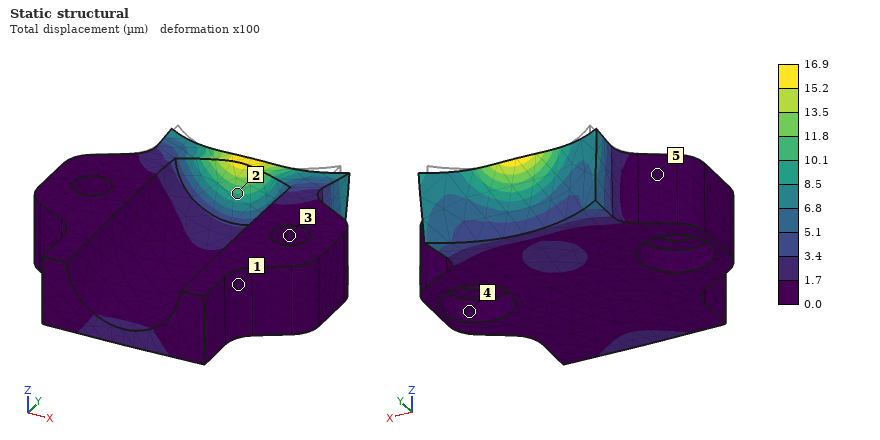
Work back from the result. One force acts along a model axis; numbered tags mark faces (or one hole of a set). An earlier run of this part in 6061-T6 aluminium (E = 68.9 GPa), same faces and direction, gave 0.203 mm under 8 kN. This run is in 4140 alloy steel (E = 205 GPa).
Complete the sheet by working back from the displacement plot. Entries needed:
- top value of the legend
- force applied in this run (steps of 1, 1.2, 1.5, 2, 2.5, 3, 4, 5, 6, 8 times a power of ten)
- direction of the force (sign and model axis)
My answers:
16.9 µm
2 kN
+Y
